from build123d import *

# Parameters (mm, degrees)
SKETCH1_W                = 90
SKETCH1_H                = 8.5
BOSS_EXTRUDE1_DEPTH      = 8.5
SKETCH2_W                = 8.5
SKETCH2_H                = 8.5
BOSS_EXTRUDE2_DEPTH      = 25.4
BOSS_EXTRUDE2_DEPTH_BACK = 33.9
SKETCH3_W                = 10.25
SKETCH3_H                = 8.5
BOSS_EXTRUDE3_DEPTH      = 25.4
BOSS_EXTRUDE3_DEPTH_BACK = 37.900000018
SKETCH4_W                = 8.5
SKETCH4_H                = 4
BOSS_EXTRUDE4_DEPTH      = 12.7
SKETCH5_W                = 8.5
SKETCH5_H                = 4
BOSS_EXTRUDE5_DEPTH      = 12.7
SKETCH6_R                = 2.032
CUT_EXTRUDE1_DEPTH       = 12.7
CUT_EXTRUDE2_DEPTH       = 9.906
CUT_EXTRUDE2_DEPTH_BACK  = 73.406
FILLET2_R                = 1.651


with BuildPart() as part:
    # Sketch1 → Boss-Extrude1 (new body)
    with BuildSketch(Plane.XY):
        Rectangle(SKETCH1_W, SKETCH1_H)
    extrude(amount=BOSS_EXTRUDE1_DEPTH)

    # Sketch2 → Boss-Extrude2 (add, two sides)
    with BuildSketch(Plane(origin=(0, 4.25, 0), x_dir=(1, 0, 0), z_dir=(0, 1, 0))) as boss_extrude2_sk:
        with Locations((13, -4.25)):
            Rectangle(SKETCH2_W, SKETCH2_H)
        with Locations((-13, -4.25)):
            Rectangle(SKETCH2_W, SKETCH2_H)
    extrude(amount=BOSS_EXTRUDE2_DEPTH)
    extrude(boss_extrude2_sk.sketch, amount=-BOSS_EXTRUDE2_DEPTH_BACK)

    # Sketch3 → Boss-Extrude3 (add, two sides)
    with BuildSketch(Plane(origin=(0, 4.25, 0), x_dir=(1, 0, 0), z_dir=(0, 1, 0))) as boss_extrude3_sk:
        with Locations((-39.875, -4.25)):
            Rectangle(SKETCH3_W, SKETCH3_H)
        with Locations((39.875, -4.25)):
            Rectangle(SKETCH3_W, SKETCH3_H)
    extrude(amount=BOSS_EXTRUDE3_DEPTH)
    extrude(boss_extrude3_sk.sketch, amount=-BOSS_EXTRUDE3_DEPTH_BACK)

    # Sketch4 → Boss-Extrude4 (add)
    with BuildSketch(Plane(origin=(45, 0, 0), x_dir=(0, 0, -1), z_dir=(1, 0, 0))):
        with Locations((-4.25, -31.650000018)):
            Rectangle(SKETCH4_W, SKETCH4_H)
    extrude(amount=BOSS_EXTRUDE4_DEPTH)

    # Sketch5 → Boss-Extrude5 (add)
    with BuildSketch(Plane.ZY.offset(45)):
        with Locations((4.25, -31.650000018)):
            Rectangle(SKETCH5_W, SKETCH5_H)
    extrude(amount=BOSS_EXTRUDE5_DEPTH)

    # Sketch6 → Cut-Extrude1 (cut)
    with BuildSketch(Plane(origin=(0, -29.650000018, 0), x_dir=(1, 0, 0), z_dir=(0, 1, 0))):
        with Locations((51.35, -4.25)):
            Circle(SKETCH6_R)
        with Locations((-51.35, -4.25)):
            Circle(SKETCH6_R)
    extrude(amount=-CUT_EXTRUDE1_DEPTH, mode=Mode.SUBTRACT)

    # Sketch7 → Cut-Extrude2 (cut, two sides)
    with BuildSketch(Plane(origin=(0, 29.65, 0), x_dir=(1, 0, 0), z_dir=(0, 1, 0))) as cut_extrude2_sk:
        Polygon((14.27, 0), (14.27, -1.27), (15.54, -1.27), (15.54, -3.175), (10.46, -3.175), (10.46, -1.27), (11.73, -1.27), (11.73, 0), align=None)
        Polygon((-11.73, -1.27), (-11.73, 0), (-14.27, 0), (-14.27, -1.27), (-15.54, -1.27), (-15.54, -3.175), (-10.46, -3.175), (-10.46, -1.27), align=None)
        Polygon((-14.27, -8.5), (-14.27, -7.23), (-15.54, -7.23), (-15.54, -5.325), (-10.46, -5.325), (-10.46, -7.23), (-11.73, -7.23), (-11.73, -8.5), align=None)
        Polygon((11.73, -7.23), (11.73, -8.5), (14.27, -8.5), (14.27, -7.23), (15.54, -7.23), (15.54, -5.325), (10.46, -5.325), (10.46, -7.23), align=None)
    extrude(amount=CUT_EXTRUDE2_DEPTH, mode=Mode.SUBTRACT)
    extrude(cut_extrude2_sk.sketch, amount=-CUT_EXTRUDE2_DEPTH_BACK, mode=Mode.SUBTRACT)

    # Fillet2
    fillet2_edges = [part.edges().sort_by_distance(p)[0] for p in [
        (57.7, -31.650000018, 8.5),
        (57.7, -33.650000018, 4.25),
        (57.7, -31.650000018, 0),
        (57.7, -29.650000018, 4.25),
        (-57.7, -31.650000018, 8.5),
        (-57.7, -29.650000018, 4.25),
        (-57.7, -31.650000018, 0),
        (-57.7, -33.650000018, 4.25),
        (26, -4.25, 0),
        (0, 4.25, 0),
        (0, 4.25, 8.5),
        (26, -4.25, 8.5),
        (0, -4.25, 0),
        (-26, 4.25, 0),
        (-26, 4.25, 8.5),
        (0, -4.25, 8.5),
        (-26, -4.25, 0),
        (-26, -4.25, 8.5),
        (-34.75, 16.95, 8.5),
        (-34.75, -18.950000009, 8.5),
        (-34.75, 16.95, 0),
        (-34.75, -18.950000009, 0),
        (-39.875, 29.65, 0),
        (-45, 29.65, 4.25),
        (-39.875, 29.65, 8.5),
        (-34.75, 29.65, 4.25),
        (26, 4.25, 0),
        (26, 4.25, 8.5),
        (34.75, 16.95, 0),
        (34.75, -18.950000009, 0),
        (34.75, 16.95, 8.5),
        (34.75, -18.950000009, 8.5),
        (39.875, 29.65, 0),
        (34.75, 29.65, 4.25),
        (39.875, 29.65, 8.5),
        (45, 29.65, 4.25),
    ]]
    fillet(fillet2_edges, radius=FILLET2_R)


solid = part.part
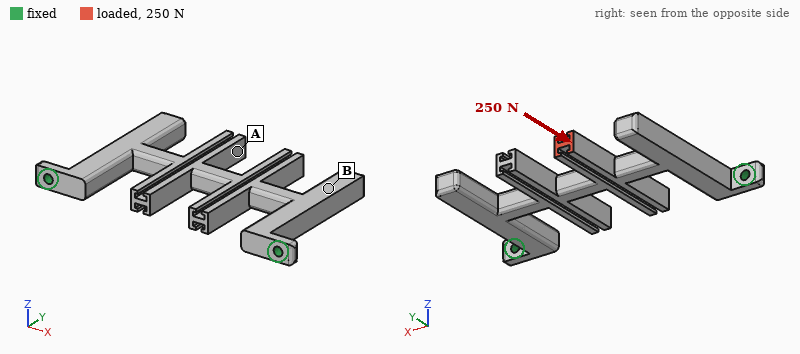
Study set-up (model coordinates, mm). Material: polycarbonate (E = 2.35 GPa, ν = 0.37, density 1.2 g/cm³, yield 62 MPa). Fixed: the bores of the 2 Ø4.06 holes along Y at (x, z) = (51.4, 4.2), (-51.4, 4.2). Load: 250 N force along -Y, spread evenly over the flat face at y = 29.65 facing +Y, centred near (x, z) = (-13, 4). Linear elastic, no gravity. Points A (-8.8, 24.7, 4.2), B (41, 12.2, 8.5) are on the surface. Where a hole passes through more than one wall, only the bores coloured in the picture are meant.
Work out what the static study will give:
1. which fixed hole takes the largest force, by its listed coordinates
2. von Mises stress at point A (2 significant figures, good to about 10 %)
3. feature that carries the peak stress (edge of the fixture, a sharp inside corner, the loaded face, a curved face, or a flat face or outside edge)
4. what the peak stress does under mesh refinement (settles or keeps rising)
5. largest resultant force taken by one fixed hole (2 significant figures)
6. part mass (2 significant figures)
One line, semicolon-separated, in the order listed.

(-51.4, 4.2); 5.4 MPa; edge of the fixture; keeps rising; 190 N; 25 g
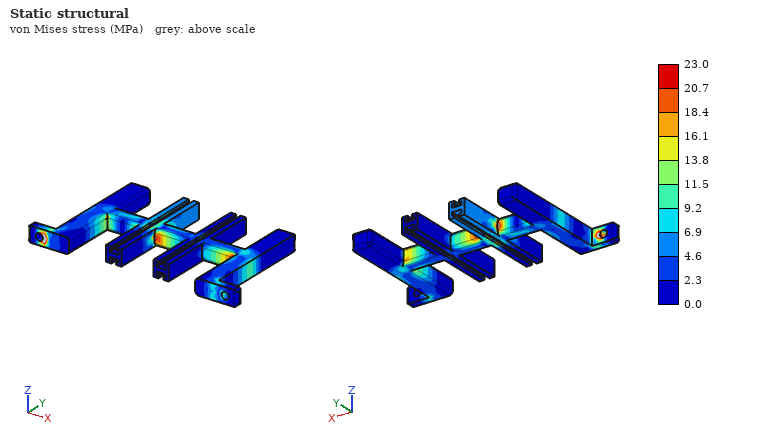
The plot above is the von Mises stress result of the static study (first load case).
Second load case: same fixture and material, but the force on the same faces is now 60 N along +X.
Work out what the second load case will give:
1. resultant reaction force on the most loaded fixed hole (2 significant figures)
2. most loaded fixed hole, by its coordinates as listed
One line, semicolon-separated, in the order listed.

54 N; (51.4, 4.2)
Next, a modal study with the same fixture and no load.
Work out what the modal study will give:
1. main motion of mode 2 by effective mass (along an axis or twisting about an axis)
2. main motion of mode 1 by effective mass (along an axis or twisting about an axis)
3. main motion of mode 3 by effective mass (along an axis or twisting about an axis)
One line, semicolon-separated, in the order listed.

twisting about Y; along Z; along X
